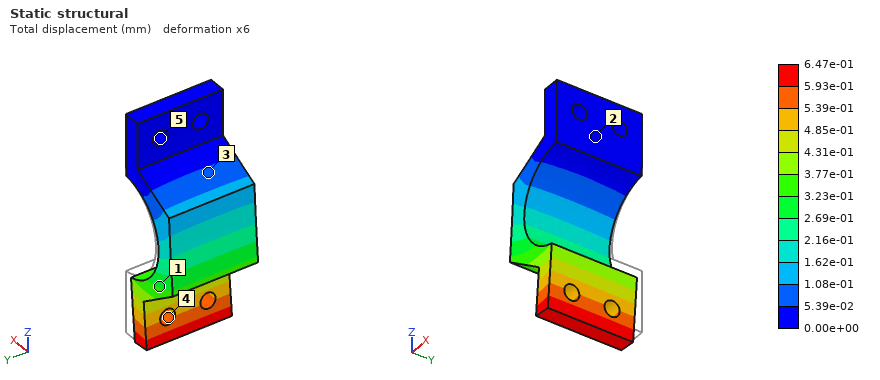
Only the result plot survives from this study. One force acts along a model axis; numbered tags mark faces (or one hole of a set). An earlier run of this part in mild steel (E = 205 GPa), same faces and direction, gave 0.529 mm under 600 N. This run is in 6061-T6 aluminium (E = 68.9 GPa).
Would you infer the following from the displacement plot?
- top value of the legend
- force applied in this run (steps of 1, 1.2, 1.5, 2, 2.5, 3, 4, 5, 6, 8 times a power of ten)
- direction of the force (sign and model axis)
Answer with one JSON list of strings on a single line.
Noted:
["6.47e-01 mm", "250 N", "-X"]
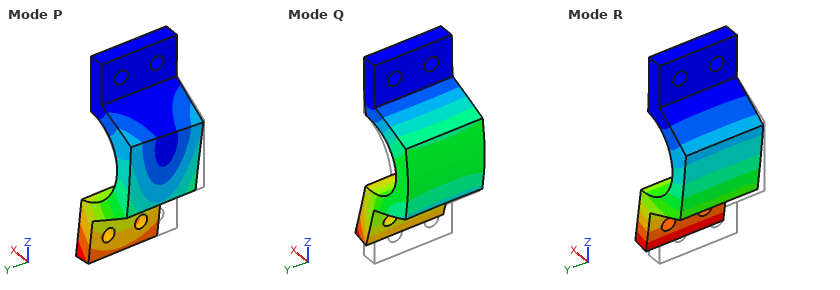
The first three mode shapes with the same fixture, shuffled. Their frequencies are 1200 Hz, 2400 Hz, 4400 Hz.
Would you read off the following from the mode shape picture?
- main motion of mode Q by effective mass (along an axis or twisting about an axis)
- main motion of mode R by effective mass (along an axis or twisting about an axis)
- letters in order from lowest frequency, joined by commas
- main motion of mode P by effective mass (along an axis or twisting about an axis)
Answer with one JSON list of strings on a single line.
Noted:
["along Z", "along X", "R, P, Q", "along Y"]
